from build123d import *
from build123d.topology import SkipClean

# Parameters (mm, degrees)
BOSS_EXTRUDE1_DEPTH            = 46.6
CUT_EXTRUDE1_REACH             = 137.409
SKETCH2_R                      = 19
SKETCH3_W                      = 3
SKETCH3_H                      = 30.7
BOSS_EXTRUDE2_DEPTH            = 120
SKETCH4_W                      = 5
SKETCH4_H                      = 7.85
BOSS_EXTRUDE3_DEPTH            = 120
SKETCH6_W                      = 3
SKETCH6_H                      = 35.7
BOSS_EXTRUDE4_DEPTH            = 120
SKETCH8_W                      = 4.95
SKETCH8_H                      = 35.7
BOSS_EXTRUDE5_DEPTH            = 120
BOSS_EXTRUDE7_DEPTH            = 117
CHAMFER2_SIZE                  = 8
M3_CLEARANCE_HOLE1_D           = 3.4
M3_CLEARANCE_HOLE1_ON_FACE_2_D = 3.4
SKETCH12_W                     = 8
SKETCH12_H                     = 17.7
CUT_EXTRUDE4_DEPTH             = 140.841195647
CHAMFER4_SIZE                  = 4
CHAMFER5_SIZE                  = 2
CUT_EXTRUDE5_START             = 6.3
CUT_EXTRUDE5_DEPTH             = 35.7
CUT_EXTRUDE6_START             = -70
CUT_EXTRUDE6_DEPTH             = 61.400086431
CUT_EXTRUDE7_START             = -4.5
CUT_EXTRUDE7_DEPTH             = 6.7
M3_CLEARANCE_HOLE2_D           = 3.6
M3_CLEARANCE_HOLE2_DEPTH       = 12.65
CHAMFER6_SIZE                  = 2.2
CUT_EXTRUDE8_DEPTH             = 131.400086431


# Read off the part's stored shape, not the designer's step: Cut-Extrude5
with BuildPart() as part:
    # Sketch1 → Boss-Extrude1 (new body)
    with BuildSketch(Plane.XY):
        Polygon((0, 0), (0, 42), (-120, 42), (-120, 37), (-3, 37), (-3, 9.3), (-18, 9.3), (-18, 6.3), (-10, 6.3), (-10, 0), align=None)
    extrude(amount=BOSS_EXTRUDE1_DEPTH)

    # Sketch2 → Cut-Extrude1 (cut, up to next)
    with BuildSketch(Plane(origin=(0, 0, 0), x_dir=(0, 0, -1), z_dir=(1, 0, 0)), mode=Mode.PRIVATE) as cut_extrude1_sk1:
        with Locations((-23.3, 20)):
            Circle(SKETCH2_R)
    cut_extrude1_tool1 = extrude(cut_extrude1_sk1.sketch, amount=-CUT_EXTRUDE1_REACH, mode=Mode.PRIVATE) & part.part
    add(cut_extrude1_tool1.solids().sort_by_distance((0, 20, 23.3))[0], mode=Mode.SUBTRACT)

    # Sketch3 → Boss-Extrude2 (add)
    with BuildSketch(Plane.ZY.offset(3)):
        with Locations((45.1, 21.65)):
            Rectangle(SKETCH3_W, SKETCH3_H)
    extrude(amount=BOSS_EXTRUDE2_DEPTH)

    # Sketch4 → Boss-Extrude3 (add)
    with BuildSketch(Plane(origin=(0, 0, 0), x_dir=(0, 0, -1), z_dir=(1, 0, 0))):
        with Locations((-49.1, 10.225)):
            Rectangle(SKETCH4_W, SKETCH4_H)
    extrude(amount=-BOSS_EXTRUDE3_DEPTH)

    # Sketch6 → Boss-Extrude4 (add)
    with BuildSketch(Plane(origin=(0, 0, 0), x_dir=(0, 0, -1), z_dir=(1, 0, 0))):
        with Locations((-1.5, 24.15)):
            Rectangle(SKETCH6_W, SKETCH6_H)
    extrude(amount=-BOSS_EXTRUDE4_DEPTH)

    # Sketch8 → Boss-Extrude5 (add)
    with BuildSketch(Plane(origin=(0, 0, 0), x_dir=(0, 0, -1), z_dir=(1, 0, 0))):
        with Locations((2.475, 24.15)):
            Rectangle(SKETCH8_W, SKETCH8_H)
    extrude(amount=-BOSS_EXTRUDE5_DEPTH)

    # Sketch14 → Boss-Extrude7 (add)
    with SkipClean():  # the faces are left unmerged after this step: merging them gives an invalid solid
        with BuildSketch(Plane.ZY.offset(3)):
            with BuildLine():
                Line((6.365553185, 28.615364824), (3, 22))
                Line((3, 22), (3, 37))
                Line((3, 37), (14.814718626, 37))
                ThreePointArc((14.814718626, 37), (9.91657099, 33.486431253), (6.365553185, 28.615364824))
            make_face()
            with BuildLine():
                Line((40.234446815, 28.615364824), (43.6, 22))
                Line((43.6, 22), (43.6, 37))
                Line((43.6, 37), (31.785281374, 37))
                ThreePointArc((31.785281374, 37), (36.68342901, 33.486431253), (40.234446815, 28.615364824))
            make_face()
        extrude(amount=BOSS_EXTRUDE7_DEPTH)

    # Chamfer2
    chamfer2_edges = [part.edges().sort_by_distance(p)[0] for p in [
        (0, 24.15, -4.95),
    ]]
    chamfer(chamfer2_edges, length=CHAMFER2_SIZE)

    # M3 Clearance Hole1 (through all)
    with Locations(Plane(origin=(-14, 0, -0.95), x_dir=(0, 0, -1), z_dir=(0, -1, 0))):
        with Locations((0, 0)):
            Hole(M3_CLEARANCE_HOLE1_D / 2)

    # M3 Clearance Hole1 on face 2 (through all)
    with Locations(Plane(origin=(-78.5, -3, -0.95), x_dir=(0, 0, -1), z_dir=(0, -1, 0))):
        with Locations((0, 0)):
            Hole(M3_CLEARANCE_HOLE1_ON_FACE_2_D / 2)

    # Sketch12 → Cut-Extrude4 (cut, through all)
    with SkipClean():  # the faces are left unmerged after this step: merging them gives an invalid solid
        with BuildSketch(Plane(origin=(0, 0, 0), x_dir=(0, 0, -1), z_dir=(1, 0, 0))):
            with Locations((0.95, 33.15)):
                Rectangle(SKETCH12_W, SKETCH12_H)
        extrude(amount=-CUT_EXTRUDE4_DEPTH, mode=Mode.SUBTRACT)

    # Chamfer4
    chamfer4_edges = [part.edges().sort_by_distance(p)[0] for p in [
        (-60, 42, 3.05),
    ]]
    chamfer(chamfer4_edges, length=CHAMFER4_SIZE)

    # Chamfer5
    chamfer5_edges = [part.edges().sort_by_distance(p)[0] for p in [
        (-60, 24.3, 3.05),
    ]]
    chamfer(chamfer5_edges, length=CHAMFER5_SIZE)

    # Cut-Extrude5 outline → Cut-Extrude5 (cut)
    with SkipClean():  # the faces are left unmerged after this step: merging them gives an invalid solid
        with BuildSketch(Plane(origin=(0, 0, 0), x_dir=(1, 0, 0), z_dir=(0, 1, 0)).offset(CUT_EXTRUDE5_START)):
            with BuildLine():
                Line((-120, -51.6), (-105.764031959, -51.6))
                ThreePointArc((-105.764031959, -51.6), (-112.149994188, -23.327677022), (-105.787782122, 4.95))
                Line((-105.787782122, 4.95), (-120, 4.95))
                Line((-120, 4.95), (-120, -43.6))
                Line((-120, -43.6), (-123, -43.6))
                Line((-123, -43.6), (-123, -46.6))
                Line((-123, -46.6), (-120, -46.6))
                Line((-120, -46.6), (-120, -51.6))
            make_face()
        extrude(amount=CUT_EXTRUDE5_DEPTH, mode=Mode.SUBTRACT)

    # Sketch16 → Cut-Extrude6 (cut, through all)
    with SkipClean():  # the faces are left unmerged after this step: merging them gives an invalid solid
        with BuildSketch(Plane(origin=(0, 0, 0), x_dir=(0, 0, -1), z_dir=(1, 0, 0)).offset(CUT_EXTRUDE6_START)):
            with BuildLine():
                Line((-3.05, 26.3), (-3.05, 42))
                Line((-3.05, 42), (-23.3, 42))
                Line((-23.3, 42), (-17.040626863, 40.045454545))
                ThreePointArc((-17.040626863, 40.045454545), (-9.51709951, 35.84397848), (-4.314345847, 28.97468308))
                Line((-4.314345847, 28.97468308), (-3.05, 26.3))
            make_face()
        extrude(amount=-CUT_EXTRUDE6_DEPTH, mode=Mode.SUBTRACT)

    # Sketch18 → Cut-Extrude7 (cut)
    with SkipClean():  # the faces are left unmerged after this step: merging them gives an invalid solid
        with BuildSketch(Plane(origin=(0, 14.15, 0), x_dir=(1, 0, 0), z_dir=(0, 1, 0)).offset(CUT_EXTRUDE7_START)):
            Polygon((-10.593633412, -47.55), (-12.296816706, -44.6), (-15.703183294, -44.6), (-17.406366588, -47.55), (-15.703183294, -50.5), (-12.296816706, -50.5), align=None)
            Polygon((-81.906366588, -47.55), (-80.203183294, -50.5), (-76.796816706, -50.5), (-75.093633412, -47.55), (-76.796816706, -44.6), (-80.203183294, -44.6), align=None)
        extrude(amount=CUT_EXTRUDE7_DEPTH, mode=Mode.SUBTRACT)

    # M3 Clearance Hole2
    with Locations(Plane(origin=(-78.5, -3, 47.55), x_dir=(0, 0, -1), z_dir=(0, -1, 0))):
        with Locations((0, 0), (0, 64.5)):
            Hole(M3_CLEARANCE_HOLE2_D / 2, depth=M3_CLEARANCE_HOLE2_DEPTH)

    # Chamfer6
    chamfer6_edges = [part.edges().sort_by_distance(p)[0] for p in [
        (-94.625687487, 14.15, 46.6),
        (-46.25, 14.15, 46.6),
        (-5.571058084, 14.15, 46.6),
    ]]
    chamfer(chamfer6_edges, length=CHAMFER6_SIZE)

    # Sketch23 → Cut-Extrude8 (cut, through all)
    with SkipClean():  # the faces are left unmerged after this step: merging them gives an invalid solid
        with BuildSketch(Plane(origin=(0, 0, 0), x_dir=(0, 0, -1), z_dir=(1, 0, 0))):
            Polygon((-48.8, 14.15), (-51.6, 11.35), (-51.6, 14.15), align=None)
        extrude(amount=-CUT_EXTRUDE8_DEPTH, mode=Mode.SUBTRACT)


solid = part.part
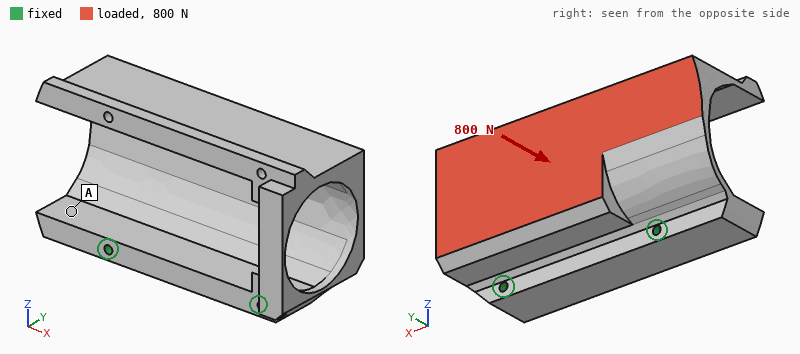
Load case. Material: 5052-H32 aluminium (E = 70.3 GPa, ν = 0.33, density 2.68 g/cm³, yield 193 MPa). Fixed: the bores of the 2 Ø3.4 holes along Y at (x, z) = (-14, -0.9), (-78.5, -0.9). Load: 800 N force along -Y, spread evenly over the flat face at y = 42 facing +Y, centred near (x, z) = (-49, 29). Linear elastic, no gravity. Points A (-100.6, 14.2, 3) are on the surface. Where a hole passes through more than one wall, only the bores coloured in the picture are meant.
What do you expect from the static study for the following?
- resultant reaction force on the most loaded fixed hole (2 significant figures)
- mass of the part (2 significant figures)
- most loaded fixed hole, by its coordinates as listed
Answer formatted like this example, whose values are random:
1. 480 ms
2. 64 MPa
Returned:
1. 440 N
2. 170 g
3. (-78.5, -0.9)
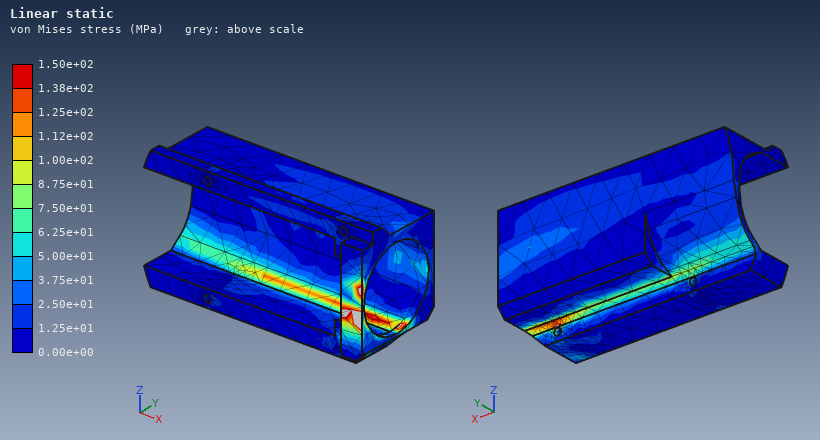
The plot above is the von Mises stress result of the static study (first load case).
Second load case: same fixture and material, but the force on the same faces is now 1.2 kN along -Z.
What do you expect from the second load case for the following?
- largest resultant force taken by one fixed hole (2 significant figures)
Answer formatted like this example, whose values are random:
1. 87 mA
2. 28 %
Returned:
1. 610 N
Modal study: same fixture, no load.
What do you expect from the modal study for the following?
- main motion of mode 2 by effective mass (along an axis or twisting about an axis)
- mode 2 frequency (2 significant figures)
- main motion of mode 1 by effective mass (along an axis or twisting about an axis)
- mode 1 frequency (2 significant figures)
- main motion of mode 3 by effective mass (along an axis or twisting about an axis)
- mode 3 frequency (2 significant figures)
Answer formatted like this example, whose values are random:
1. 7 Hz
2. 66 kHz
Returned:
1. along X
2. 1200 Hz
3. along Y
4. 610 Hz
5. along Z
6. 1700 Hz
